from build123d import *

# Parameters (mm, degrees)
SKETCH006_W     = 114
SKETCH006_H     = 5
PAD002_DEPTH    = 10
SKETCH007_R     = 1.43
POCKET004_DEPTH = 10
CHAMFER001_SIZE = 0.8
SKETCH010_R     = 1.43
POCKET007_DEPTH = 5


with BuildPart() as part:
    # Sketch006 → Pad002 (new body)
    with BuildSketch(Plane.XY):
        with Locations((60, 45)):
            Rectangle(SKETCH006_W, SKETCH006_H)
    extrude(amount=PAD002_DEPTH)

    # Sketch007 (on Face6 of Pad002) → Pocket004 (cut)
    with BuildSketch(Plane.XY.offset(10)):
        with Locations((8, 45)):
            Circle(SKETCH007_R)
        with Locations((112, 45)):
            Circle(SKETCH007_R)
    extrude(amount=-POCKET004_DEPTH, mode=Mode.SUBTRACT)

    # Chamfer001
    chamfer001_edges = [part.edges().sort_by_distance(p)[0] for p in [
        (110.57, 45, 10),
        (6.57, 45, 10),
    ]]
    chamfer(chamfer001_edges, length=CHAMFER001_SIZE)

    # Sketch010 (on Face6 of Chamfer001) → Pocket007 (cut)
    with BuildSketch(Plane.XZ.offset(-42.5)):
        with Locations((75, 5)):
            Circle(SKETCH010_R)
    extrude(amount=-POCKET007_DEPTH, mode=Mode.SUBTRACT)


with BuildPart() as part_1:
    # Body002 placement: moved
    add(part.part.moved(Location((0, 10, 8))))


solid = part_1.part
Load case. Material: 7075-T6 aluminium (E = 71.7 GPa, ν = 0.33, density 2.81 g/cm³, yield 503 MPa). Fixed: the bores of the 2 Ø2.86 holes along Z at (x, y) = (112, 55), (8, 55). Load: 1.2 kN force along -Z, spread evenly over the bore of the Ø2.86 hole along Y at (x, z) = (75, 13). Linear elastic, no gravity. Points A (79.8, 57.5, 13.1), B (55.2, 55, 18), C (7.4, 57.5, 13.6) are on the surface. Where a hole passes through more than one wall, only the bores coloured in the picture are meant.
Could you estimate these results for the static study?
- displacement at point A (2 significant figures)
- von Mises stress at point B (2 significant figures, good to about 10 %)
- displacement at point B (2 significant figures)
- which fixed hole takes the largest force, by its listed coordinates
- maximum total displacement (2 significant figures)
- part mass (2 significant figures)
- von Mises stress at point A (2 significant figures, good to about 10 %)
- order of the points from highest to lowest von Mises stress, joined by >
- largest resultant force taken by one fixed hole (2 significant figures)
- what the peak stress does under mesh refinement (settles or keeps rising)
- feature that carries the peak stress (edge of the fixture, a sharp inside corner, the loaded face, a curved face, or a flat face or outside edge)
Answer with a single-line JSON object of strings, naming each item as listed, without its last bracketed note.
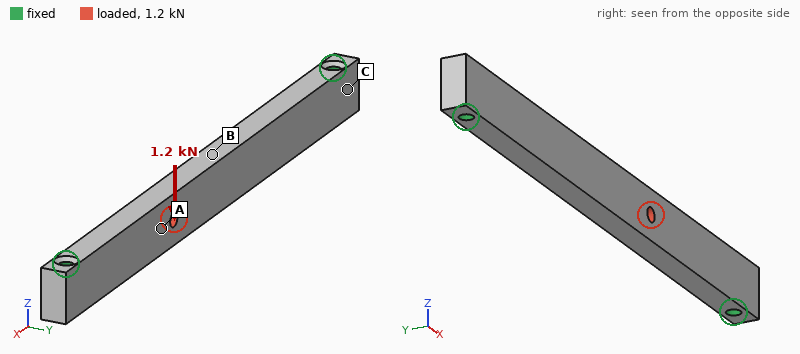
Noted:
{"displacement at point A": "0.18 mm", "von Mises stress at point B": "73 MPa", "displacement at point B": "0.19 mm", "which fixed hole takes the largest force, by its listed coordinates": "(112, 55)", "maximum total displacement": "0.21 mm", "part mass": "16 g", "von Mises stress at point A": "45 MPa", "order of the points from highest to lowest von Mises stress, joined by >": "B > A > C", "largest resultant force taken by one fixed hole": "850 N", "what the peak stress does under mesh refinement": "keeps rising", "feature that carries the peak stress": "edge of the fixture"}
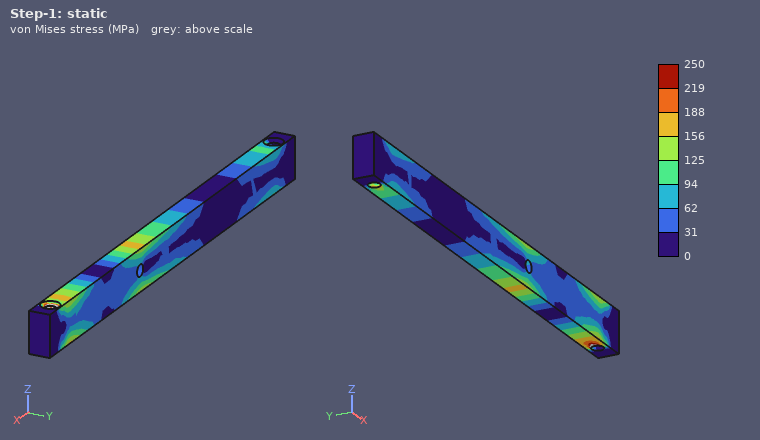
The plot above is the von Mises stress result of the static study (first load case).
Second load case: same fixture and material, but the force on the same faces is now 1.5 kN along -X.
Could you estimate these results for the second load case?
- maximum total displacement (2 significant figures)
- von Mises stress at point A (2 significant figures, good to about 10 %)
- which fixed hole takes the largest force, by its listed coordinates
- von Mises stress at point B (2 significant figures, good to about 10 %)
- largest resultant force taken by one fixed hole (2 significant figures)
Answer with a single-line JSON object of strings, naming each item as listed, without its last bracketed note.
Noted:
{"maximum total displacement": "11 µm", "von Mises stress at point A": "26 MPa", "which fixed hole takes the largest force, by its listed coordinates": "(112, 55)", "von Mises stress at point B": "11 MPa", "largest resultant force taken by one fixed hole": "970 N"}
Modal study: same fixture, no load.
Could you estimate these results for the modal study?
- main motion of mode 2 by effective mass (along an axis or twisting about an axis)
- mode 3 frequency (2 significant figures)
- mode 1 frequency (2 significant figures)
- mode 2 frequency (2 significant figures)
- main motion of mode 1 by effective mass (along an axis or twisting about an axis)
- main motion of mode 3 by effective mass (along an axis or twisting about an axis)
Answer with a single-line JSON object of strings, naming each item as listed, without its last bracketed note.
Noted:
{"main motion of mode 2 by effective mass": "along Z", "mode 3 frequency": "6400 Hz", "mode 1 frequency": "2400 Hz", "mode 2 frequency": "4600 Hz", "main motion of mode 1 by effective mass": "along Y", "main motion of mode 3 by effective mass": "twisting about Z"}
